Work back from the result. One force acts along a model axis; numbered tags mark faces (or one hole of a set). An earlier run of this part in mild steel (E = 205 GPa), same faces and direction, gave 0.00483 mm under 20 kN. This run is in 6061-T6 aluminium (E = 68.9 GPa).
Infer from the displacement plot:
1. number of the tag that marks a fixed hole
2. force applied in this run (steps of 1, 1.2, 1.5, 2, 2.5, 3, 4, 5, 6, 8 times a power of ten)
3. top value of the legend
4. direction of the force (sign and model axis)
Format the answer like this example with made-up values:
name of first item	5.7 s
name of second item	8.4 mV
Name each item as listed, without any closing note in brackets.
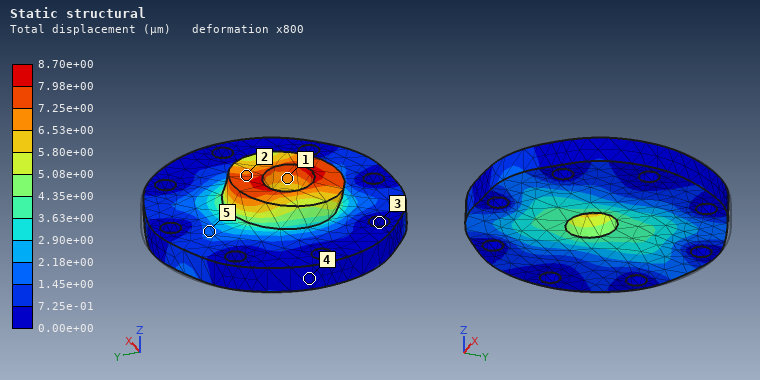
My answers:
number of the tag that marks a fixed hole	3
force applied in this run	12 kN
top value of the legend	8.70e+00 µm
direction of the force	-Y
